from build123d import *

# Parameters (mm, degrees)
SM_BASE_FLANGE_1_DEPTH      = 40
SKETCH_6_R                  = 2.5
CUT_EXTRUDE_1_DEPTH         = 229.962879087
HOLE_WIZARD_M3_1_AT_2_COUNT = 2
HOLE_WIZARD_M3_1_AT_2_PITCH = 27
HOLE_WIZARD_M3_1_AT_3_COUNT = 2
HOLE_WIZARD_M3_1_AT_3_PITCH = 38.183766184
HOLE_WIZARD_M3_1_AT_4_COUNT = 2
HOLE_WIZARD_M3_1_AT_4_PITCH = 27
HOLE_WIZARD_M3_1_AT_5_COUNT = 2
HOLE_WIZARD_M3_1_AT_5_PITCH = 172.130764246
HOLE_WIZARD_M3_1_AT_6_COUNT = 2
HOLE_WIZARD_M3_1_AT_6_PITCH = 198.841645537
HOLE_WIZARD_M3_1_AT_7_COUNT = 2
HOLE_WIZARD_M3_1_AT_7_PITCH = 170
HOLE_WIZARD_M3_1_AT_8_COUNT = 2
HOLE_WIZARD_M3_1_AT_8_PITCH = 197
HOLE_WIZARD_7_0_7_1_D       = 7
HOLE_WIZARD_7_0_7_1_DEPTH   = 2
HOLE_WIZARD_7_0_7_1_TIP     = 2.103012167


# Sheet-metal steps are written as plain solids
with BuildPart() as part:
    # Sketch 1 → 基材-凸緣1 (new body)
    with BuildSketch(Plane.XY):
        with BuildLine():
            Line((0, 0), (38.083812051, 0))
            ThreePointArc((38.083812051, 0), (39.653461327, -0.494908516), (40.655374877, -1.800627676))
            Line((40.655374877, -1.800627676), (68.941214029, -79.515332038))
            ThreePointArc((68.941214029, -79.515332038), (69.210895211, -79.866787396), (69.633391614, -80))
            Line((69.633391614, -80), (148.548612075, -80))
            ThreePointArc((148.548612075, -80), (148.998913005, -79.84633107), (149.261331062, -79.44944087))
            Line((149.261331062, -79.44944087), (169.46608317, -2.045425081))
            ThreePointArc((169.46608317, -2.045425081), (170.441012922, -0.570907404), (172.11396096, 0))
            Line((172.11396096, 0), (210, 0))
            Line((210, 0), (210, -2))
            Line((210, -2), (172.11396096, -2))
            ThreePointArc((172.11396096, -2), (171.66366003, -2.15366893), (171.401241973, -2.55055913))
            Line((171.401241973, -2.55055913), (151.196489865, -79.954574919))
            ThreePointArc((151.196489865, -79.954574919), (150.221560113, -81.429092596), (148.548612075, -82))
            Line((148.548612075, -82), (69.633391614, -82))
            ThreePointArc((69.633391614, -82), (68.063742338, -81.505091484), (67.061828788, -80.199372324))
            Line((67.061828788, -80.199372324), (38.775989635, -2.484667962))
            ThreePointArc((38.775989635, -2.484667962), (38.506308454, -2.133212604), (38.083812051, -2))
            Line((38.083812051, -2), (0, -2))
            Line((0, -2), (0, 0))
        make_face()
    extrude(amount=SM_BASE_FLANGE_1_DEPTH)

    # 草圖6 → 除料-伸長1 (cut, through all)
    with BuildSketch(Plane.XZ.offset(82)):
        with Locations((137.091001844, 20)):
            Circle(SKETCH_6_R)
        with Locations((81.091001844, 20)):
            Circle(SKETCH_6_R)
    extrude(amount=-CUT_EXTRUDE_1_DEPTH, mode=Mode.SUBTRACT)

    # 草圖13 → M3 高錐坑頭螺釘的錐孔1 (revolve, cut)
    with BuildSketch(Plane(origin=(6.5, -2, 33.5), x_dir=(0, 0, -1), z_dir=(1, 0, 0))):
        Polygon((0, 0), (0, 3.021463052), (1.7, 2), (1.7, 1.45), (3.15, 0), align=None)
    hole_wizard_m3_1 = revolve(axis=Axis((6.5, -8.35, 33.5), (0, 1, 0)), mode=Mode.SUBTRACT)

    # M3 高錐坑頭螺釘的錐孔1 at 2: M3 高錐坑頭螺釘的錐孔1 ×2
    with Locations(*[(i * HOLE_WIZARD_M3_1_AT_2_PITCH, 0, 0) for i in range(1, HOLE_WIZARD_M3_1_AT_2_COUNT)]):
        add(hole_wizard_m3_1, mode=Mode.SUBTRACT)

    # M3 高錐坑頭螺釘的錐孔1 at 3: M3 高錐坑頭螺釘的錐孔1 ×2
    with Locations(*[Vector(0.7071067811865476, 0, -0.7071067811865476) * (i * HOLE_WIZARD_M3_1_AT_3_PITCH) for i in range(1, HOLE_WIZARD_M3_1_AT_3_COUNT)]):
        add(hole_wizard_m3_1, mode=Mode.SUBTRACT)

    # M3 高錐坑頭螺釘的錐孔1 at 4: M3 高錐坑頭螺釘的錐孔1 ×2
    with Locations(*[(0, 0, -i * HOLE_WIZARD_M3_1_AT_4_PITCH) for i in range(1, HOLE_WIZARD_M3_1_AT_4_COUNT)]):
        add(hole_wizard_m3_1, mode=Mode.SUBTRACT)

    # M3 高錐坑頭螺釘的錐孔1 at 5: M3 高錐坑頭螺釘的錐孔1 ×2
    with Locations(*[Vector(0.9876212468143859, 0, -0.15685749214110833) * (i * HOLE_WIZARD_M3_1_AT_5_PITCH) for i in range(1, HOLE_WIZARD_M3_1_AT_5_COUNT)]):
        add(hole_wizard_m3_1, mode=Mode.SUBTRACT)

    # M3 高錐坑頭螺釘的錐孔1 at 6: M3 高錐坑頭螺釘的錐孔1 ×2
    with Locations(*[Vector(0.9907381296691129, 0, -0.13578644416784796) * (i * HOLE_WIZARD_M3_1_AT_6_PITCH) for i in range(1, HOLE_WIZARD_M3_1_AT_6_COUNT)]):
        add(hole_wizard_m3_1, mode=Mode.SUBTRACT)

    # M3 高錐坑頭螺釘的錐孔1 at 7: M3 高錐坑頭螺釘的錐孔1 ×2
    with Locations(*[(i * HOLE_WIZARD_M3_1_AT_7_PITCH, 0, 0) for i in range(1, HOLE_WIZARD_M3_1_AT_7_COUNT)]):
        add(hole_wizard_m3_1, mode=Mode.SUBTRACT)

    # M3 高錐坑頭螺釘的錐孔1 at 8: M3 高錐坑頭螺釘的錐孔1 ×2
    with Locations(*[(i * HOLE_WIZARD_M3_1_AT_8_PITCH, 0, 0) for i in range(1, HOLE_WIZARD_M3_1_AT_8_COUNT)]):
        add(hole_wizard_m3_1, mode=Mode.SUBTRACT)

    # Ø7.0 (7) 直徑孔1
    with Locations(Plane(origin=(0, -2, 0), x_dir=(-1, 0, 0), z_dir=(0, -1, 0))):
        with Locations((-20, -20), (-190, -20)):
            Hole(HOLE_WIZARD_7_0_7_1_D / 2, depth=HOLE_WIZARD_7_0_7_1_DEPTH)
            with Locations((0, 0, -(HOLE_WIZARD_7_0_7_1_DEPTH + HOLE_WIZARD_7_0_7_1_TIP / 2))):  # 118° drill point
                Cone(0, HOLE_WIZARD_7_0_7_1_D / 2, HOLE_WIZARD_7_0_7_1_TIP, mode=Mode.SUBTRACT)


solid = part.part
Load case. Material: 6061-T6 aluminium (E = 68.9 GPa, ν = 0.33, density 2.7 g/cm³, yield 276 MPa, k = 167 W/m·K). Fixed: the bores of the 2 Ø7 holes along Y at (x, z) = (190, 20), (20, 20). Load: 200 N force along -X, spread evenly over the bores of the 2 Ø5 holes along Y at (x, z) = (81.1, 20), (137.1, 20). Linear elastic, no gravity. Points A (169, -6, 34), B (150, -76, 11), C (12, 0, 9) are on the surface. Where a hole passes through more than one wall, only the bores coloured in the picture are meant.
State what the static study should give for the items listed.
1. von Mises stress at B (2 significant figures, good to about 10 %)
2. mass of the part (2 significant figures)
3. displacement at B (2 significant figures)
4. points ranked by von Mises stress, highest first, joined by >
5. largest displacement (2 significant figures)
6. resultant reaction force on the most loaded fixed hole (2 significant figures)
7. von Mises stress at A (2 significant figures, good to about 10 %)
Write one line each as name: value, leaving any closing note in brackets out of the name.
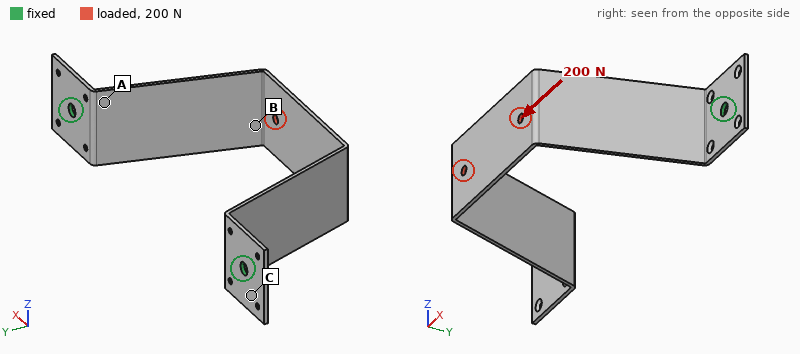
von Mises stress at B: 110 MPa
mass of the part: 69 g
displacement at B: 2.6 mm
points ranked by von Mises stress, highest first, joined by >: B > A > C
largest displacement: 2.7 mm
resultant reaction force on the most loaded fixed hole: 130 N
von Mises stress at A: 70 MPa
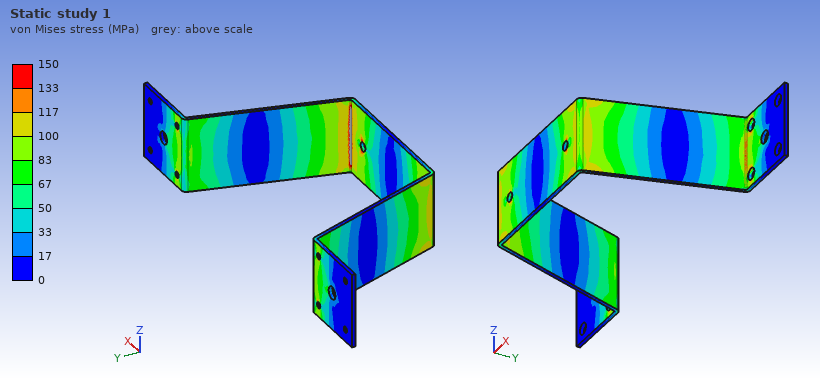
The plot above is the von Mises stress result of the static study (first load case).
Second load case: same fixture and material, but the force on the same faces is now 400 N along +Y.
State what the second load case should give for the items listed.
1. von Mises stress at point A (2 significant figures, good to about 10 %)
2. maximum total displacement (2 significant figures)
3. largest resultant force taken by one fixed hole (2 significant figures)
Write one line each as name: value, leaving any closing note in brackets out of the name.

von Mises stress at point A: 37 MPa
maximum total displacement: 0.60 mm
largest resultant force taken by one fixed hole: 230 N
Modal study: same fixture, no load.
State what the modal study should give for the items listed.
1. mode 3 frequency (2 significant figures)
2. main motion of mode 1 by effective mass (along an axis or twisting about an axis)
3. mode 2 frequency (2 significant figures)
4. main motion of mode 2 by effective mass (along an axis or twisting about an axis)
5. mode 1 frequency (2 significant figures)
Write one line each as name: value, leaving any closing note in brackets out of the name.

mode 3 frequency: 440 Hz
main motion of mode 1 by effective mass: along Z
mode 2 frequency: 240 Hz
main motion of mode 2 by effective mass: along X
mode 1 frequency: 230 Hz
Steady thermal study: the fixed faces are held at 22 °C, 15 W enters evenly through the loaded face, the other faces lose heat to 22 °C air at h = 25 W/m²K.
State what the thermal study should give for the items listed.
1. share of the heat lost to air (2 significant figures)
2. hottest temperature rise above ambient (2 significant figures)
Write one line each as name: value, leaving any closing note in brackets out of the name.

share of the heat lost to air: 68 %
hottest temperature rise above ambient: 35 K
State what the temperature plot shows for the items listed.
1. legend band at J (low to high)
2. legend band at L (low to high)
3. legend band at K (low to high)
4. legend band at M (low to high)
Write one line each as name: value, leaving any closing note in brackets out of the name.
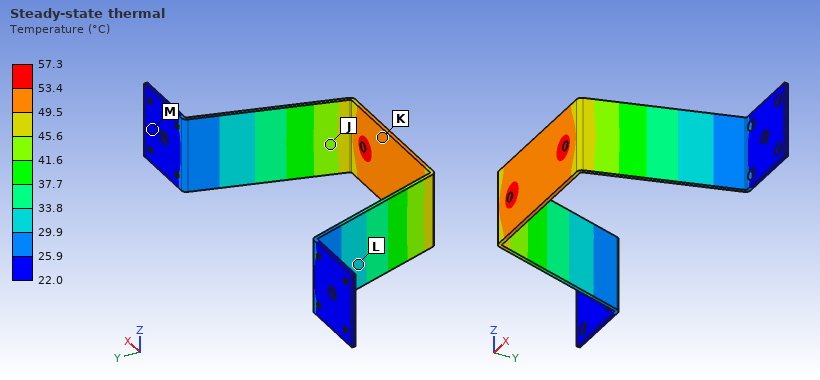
legend band at J: 41.6 to 45.6 °C
legend band at L: 29.9 to 33.8 °C
legend band at K: 49.5 to 53.4 °C
legend band at M: 22.0 to 25.9 °C
